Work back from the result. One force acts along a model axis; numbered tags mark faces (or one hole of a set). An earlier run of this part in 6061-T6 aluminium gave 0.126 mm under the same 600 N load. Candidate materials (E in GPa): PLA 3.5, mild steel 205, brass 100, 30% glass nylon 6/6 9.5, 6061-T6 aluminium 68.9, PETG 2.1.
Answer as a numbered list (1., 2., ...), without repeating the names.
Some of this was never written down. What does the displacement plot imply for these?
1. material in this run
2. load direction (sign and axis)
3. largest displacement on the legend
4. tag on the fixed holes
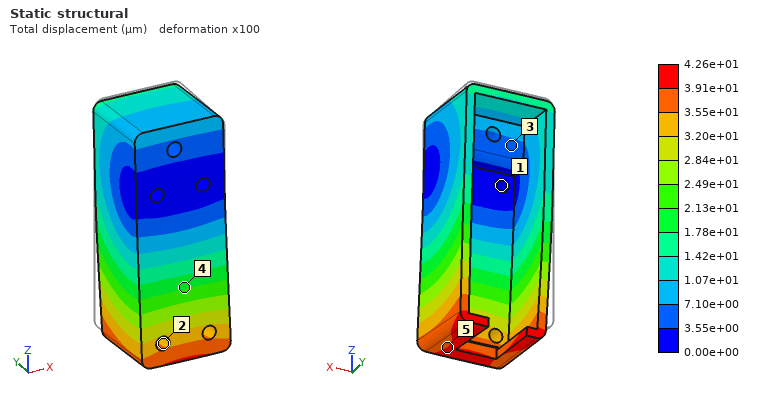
1. mild steel
2. -Y
3. 4.26e+01 µm
4. 1
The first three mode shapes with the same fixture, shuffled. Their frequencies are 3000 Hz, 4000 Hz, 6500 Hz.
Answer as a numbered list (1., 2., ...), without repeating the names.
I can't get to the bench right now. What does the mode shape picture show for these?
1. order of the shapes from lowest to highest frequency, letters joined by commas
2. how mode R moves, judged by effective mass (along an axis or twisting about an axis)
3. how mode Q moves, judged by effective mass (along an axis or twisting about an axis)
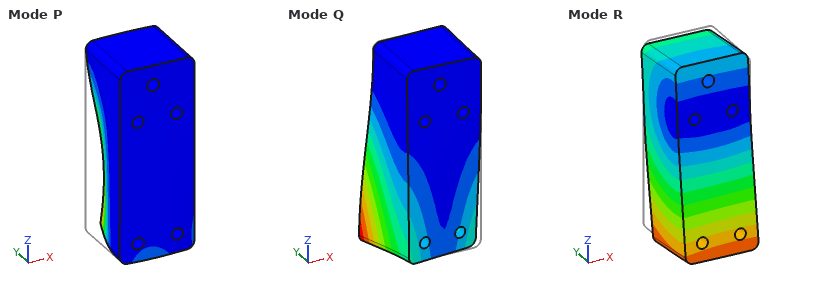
1. R, Q, P
2. along Y
3. along X
